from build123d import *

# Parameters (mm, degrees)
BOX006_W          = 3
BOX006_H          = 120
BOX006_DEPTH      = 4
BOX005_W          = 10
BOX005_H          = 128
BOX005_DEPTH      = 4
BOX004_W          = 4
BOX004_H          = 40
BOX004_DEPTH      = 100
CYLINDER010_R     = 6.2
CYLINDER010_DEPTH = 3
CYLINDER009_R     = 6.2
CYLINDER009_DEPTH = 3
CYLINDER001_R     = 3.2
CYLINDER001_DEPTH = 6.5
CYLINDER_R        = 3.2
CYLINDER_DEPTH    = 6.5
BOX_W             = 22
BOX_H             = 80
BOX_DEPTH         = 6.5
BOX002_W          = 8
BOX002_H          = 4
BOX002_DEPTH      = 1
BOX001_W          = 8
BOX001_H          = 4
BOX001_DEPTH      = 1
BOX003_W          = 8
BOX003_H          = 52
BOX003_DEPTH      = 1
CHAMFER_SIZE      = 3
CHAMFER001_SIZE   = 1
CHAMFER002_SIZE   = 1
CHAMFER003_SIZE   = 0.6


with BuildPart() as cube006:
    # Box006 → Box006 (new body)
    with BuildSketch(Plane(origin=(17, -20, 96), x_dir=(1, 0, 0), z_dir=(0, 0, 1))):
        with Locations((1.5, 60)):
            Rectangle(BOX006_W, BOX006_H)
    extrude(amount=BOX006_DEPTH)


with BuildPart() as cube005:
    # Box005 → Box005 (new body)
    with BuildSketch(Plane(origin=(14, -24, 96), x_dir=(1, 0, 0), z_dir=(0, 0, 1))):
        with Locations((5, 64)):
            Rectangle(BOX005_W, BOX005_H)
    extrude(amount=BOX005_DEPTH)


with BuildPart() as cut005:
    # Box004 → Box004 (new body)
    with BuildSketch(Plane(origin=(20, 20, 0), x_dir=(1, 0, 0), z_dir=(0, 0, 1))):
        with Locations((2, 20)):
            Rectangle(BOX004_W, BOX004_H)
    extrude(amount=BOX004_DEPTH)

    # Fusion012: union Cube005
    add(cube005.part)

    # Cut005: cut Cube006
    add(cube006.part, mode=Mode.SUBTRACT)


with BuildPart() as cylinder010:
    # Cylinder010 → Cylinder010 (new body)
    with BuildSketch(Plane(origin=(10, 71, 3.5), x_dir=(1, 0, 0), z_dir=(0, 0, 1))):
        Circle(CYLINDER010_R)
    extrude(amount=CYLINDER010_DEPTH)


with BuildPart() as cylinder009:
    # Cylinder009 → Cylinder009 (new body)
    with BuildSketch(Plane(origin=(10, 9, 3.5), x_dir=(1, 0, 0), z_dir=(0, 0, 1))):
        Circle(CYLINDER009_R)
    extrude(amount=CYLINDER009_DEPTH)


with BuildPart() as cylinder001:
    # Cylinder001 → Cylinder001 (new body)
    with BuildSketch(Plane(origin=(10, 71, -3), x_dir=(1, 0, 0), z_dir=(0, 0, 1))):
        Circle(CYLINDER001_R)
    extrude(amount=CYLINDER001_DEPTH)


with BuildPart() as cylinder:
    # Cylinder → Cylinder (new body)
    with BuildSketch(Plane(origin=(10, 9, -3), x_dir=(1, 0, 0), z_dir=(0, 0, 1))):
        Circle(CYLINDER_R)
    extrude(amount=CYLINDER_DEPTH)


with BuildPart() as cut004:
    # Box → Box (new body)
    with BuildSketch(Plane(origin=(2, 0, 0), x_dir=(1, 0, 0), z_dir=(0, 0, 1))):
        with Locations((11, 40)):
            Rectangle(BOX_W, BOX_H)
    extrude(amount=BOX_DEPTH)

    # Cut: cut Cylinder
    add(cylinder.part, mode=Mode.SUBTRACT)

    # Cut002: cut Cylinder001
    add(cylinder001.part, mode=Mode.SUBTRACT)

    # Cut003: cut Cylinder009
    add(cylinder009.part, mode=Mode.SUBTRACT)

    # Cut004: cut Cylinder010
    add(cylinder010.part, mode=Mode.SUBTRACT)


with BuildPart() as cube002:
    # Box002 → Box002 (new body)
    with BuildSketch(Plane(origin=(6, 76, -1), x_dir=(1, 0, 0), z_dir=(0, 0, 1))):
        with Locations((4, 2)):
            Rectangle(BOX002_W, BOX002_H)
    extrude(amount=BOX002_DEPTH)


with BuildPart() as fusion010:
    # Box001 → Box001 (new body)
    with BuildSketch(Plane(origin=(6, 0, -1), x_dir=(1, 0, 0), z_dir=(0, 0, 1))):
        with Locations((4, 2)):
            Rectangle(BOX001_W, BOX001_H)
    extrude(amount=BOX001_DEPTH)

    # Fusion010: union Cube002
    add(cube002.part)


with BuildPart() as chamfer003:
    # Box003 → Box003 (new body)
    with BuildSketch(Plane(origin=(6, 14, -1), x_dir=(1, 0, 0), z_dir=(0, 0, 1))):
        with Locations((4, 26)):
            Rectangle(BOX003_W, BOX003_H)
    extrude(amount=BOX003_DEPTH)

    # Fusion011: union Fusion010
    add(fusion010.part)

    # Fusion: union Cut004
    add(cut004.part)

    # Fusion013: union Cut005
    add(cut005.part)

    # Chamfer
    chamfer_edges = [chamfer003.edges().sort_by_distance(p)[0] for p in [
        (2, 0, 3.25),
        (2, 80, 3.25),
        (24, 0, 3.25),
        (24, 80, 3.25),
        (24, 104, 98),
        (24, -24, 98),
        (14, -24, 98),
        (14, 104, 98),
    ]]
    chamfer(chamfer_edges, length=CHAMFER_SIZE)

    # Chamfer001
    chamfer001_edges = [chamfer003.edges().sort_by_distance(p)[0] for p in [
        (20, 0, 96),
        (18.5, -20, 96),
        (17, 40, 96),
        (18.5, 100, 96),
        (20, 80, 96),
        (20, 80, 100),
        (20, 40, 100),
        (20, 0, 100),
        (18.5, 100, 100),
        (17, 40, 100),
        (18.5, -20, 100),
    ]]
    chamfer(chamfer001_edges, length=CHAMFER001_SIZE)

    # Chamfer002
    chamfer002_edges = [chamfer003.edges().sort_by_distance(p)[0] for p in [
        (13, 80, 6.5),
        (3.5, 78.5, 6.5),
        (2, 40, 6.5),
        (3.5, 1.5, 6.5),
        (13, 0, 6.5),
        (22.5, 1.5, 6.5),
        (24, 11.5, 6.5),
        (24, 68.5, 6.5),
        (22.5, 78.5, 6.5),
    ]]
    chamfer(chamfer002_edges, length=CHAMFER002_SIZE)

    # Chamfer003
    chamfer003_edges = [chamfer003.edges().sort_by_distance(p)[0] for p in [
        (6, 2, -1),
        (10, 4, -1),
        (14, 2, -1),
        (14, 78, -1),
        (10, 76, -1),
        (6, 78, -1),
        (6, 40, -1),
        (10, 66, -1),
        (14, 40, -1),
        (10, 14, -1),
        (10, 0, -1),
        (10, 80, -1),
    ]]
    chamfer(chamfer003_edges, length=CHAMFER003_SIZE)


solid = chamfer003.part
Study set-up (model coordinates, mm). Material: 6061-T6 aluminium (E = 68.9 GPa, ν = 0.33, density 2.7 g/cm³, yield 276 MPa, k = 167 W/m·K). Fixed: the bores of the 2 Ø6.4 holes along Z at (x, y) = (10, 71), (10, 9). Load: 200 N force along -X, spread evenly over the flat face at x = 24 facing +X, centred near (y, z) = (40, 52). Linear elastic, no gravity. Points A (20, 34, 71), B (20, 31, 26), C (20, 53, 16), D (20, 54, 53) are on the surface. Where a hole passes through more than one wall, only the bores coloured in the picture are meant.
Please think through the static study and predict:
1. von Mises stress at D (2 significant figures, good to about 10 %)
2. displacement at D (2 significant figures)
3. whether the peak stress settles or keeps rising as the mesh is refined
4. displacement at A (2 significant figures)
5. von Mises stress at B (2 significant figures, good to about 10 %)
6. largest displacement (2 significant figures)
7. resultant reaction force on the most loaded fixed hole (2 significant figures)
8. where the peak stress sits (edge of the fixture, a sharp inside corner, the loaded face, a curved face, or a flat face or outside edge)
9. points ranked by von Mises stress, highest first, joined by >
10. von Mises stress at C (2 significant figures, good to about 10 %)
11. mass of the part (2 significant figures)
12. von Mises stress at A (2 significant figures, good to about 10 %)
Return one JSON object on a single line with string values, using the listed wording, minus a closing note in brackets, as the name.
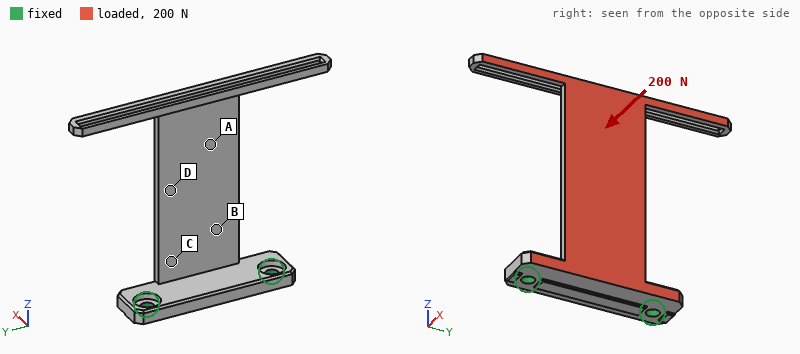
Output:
{"von Mises stress at D": "25 MPa", "displacement at D": "0.67 mm", "whether the peak stress settles or keeps rising as the mesh is refined": "keeps rising", "displacement at A": "1.1 mm", "von Mises stress at B": "52 MPa", "largest displacement": "1.8 mm", "resultant reaction force on the most loaded fixed hole": "140 N", "where the peak stress sits": "edge of the fixture", "points ranked by von Mises stress, highest first, joined by >": "C > B > D > A", "von Mises stress at C": "65 MPa", "mass of the part": "77 g", "von Mises stress at A": "11 MPa"}
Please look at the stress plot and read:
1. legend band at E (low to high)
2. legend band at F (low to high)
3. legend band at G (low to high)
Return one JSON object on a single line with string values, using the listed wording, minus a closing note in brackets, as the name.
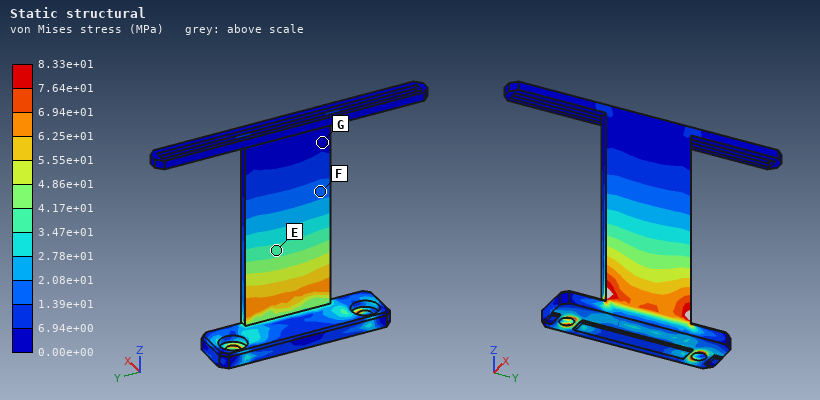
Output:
{"legend band at E": "3.47e+01 to 4.17e+01 MPa", "legend band at F": "1.39e+01 to 2.08e+01 MPa", "legend band at G": "0.00e+00 to 6.94e+00 MPa"}
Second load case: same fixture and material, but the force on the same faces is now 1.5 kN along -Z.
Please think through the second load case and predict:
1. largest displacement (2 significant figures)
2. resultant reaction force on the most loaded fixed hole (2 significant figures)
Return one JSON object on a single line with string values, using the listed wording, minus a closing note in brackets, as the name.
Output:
{"largest displacement": "1.1 mm", "resultant reaction force on the most loaded fixed hole": "860 N"}
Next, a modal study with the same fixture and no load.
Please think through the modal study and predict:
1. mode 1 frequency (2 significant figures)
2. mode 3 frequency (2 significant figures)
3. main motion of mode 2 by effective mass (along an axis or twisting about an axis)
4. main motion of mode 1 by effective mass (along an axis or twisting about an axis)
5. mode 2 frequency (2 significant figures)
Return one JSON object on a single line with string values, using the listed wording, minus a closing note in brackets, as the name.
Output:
{"mode 1 frequency": "250 Hz", "mode 3 frequency": "840 Hz", "main motion of mode 2 by effective mass": "twisting about Z", "main motion of mode 1 by effective mass": "along X", "mode 2 frequency": "560 Hz"}
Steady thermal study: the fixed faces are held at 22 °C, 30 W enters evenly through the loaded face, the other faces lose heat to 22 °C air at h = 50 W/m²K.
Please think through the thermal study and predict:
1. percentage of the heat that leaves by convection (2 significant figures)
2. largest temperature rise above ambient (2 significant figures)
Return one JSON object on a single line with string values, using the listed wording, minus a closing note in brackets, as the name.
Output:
{"percentage of the heat that leaves by convection": "36 %", "largest temperature rise above ambient": "38 K"}
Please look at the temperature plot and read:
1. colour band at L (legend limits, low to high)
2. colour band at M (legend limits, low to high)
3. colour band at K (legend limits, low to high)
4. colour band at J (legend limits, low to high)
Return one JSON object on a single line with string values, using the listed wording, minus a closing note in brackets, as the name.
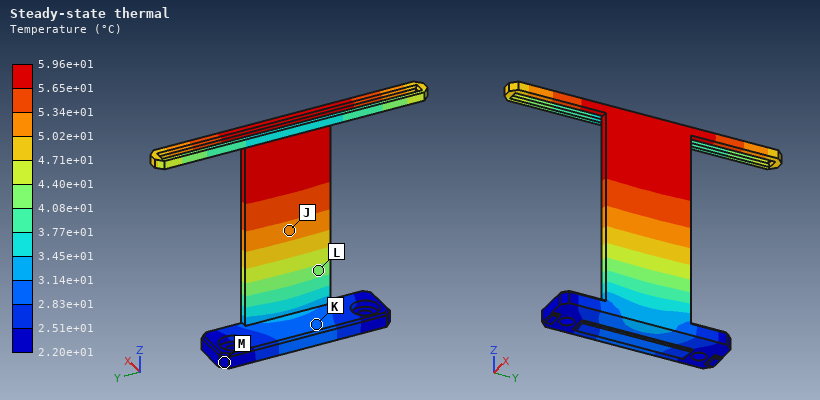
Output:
{"colour band at L": "4.08e+01 to 4.40e+01 °C", "colour band at M": "2.20e+01 to 2.51e+01 °C", "colour band at K": "2.83e+01 to 3.14e+01 °C", "colour band at J": "5.02e+01 to 5.34e+01 °C"}
